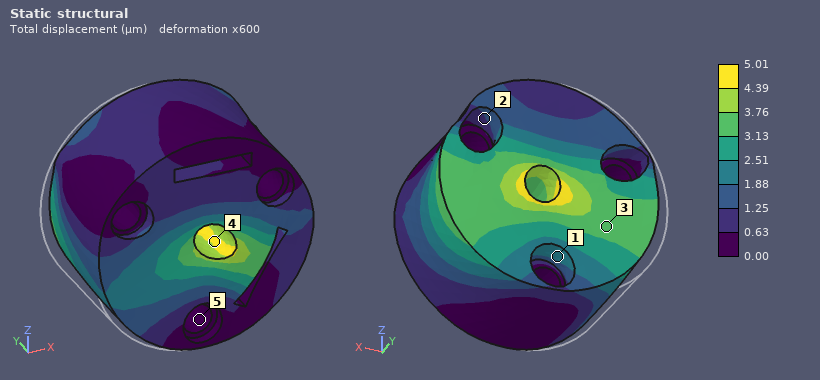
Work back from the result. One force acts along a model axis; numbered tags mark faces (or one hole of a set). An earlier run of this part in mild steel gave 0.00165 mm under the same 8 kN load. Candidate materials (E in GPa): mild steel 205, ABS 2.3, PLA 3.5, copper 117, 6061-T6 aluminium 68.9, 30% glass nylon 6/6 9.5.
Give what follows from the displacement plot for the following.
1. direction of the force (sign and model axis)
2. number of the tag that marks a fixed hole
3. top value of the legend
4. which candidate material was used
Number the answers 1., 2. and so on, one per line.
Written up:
1. +X
2. 5
3. 5.01 µm
4. 6061-T6 aluminium
